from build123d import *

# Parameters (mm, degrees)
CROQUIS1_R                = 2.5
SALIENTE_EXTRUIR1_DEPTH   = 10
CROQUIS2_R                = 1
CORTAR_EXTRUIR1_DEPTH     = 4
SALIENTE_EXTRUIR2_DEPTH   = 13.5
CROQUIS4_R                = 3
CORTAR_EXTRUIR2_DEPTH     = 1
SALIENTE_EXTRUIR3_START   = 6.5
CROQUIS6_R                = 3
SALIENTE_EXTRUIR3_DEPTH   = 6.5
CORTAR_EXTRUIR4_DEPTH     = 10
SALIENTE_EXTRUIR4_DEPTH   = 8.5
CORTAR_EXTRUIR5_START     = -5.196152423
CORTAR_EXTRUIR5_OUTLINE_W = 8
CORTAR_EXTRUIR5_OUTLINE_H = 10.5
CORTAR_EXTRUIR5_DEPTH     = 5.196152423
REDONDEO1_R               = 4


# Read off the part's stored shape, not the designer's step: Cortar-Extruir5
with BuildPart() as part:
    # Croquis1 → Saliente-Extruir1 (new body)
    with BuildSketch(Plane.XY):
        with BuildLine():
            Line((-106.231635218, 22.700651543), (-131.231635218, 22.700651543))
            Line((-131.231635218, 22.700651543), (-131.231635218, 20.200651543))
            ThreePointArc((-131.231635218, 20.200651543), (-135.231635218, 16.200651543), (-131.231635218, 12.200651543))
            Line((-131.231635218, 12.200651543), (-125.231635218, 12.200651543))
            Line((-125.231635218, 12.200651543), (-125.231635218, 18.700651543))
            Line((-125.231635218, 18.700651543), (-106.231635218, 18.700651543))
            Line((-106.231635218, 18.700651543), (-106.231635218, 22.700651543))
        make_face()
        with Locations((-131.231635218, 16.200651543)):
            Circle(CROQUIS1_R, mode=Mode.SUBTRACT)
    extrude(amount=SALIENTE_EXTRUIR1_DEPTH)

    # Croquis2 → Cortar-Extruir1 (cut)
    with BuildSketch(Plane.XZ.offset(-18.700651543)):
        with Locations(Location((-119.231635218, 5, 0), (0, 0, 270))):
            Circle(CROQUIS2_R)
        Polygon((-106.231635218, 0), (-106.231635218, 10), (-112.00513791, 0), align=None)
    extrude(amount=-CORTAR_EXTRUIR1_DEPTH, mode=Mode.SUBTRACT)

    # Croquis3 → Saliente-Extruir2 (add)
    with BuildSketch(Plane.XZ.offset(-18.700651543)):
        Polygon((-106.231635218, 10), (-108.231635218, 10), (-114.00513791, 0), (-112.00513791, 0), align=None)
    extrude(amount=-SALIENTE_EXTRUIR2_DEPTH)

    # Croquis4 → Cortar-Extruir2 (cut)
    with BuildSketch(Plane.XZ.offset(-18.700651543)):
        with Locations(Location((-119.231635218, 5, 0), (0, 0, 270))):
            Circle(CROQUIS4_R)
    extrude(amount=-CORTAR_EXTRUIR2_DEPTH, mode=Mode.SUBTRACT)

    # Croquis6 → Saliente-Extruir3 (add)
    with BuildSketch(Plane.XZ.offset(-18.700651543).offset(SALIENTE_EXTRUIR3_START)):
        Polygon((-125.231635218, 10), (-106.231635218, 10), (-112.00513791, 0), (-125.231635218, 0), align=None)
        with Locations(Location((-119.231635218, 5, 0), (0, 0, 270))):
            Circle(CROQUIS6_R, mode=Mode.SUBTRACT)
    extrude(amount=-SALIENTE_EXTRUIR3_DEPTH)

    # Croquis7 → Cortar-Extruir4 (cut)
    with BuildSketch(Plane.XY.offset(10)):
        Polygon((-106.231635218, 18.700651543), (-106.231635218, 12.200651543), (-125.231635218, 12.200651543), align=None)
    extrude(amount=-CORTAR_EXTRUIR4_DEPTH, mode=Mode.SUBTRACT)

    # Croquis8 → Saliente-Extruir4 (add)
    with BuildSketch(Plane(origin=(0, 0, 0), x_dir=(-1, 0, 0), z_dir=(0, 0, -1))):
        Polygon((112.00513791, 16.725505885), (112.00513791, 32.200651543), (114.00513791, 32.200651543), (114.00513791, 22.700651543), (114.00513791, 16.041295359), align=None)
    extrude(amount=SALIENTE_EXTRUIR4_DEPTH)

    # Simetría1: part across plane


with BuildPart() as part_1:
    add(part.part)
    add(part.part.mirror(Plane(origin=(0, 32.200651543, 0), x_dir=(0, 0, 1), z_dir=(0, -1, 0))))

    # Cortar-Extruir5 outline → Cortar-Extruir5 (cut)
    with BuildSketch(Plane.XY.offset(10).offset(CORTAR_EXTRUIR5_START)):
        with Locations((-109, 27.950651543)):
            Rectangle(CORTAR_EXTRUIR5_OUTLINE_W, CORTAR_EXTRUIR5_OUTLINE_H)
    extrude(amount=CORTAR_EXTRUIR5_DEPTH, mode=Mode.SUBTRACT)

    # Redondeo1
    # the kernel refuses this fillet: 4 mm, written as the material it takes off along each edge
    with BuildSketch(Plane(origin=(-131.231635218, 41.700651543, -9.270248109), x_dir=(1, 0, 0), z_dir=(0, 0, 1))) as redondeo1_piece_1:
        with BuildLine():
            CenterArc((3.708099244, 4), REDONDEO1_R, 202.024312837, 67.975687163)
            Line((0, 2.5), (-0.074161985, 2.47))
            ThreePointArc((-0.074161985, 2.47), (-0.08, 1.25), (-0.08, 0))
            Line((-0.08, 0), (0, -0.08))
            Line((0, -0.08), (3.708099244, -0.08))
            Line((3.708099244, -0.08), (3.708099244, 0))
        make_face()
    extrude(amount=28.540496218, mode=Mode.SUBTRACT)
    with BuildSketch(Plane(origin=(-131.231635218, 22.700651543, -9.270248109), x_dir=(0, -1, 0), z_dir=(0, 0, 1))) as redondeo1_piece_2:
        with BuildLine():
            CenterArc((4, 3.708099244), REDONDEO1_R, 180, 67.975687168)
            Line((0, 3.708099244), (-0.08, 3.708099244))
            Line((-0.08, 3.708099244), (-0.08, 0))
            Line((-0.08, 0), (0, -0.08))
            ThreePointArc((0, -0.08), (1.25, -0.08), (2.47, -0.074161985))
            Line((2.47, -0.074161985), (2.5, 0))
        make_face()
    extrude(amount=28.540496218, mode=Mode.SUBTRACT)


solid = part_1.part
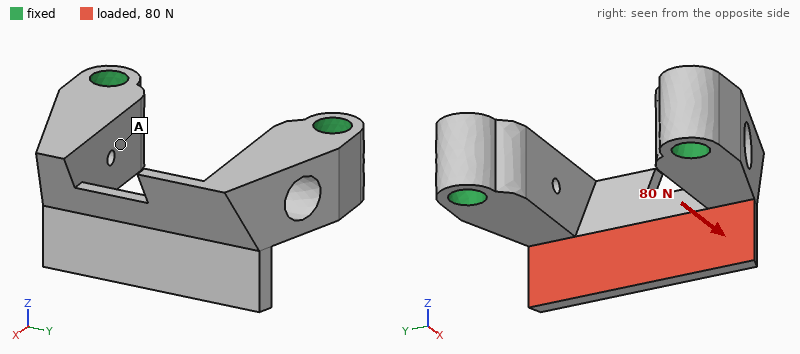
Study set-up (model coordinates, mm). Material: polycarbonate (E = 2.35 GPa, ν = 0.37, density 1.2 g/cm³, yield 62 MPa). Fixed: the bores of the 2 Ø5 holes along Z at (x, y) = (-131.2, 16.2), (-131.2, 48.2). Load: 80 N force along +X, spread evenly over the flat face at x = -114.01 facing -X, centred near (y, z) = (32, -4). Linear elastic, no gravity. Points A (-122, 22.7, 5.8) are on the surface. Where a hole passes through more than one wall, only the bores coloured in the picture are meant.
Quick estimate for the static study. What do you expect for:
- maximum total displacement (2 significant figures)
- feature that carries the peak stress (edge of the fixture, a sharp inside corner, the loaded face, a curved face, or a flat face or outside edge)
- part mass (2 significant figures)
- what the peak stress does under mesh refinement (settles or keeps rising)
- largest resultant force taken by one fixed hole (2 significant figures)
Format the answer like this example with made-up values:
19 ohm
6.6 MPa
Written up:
0.46 mm
a sharp inside corner
5.1 g
keeps rising
42 N
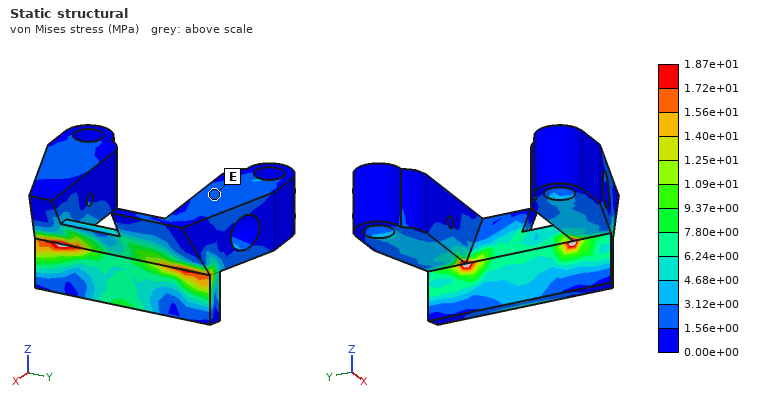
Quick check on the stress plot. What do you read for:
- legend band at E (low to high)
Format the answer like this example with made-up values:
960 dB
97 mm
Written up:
1.56e+00 to 3.12e+00 MPa
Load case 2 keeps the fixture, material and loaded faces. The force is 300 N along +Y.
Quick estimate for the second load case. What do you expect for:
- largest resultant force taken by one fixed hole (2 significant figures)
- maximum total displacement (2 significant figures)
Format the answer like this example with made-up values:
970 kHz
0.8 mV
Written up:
160 N
0.56 mm
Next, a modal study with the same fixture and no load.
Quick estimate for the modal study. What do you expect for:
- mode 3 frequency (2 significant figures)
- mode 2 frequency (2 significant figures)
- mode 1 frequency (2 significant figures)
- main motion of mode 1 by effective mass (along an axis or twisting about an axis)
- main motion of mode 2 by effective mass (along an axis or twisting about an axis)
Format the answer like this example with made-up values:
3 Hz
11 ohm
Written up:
4100 Hz
3400 Hz
3100 Hz
along Z
along Y
